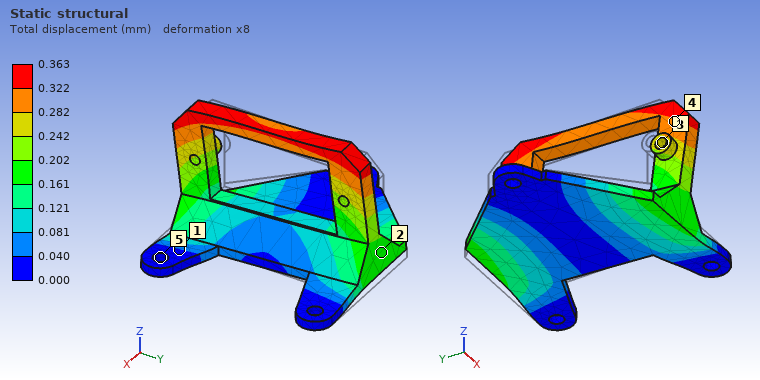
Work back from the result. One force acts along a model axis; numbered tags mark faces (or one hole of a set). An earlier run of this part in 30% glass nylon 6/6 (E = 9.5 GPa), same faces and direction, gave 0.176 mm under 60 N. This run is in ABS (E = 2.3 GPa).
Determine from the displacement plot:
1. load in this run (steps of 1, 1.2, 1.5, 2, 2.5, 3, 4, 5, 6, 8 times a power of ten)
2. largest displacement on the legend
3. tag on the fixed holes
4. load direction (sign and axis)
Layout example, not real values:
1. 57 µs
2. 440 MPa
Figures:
1. 30 N
2. 0.363 mm
3. 5
4. -Y
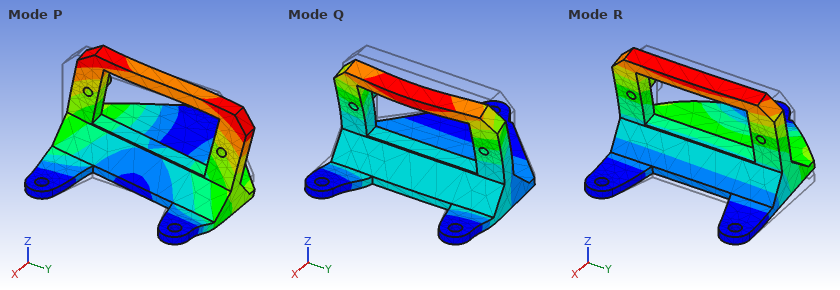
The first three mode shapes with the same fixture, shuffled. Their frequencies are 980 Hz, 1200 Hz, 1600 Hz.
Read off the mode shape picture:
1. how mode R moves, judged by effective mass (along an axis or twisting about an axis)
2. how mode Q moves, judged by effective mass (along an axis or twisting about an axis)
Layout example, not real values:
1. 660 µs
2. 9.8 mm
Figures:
1. along Z
2. along Z
